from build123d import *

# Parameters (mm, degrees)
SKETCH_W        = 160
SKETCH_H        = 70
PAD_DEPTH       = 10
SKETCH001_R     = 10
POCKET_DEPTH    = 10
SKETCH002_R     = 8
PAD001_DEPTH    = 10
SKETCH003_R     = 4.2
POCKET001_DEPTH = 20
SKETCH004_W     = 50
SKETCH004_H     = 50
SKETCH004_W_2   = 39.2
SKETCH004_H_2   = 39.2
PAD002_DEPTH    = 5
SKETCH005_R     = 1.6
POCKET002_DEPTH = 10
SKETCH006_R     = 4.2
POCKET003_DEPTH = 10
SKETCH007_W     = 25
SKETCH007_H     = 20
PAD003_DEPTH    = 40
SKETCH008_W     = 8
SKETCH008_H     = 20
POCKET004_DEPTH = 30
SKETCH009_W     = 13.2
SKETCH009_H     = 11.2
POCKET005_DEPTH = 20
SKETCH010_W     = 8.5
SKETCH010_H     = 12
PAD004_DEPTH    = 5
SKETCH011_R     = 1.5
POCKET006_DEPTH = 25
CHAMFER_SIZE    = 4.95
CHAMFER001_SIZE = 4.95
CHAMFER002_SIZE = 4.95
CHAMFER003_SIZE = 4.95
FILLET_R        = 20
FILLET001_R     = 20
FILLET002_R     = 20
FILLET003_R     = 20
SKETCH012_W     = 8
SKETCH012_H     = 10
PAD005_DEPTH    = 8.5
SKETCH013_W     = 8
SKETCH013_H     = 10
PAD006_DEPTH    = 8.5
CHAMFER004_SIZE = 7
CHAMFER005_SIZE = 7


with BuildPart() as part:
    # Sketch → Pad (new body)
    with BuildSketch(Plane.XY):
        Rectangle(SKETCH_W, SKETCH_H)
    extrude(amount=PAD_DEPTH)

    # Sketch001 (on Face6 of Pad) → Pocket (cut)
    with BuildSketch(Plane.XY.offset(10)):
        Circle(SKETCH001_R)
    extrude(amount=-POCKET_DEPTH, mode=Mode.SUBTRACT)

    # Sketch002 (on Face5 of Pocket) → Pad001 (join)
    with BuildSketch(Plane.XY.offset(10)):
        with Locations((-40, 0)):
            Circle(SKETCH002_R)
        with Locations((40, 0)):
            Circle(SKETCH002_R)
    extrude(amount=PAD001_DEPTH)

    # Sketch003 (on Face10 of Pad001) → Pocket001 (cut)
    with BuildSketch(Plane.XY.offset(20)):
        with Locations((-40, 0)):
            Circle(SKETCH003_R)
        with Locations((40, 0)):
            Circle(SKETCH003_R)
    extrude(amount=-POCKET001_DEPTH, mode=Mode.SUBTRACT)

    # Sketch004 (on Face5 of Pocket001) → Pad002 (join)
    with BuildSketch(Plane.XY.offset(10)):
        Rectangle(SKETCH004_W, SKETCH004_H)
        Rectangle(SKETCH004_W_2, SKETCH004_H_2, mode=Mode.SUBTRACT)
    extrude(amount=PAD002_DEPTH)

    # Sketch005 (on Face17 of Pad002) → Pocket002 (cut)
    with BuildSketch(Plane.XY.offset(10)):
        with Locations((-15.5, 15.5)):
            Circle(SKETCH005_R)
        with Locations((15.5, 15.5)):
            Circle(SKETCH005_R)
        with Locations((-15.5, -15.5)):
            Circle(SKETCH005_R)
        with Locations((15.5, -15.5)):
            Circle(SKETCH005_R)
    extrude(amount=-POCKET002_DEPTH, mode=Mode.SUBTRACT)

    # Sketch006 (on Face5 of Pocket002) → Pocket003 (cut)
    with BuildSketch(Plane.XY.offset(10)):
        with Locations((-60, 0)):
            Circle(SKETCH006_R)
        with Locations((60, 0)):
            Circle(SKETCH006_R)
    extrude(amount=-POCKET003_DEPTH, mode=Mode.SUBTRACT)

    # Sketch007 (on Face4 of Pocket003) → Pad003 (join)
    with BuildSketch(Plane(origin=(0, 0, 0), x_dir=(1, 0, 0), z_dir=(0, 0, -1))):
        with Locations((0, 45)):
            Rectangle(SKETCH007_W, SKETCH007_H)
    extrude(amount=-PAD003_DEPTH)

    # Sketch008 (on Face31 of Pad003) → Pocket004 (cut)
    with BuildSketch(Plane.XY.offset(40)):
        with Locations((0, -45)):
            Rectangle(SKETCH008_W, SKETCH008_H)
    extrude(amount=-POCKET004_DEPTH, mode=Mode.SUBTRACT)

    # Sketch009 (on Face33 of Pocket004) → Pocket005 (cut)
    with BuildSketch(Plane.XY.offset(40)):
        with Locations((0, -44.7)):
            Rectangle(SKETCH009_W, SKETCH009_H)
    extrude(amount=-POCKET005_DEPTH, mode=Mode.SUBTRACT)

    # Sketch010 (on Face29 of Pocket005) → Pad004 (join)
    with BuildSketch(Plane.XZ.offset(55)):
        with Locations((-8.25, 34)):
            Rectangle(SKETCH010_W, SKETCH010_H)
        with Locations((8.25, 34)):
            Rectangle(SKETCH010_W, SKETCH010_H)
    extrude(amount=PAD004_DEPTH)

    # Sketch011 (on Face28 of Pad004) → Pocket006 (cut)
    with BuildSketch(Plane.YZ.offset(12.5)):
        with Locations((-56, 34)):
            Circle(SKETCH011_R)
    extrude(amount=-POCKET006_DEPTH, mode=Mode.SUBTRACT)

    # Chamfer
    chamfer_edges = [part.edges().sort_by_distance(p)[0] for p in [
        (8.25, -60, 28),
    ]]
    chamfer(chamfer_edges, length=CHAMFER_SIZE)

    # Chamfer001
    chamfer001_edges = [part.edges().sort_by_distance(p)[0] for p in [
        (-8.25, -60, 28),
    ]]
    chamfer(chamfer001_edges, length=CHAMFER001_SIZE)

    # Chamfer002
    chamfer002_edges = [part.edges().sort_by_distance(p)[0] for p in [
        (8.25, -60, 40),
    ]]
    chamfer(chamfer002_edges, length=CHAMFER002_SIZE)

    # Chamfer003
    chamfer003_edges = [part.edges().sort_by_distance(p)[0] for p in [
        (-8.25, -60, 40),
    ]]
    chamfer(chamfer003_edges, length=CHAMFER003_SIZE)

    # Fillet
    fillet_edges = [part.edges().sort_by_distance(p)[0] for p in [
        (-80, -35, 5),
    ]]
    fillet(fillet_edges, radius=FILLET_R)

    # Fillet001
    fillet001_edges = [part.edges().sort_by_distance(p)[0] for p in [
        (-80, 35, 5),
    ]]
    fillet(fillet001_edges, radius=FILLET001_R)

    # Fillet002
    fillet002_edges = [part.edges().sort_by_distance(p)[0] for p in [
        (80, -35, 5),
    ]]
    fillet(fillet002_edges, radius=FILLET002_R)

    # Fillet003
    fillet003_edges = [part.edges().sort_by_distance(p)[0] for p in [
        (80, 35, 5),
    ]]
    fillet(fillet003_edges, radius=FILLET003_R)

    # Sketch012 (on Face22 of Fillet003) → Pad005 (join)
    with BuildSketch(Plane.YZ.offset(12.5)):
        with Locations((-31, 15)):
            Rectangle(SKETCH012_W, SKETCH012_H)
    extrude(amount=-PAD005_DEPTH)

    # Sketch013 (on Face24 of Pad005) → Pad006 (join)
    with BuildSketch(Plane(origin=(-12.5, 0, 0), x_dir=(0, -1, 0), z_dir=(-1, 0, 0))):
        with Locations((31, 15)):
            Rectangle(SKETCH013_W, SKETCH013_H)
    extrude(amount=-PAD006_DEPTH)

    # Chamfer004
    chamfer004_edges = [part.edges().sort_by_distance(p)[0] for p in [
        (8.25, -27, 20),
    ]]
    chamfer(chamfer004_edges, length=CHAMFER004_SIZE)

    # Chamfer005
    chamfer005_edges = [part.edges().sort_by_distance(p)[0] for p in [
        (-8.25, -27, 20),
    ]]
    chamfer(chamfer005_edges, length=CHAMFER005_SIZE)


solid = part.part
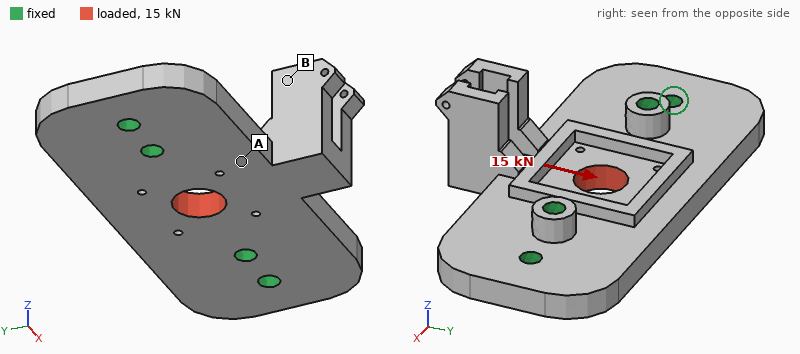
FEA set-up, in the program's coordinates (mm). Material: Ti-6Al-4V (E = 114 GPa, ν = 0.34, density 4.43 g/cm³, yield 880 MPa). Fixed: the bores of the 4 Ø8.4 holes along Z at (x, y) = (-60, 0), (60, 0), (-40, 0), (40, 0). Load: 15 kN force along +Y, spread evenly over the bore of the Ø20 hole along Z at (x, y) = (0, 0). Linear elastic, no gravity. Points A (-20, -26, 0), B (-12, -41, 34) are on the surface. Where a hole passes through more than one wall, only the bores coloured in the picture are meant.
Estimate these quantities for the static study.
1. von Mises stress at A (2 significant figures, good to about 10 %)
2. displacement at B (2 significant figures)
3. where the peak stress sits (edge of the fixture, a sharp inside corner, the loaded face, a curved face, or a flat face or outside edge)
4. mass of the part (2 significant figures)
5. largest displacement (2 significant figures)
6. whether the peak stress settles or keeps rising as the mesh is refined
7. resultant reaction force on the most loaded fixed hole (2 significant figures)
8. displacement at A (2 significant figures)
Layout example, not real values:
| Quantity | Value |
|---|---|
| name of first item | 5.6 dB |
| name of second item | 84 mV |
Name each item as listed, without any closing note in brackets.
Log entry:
| Quantity | Value |
|---|---|
| von Mises stress at A | 18 MPa |
| displacement at B | 10 µm |
| where the peak stress sits | edge of the fixture |
| mass of the part | 560 g |
| largest displacement | 15 µm |
| whether the peak stress settles or keeps rising as the mesh is refined | keeps rising |
| resultant reaction force on the most loaded fixed hole | 8.4 kN |
| displacement at A | 9.1 µm |
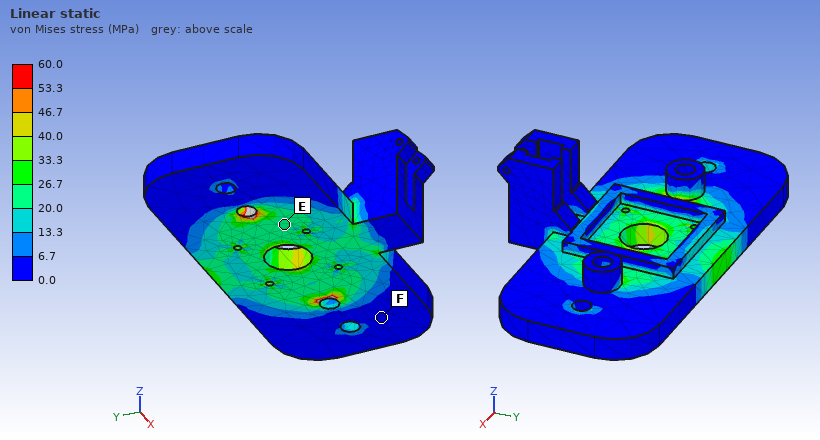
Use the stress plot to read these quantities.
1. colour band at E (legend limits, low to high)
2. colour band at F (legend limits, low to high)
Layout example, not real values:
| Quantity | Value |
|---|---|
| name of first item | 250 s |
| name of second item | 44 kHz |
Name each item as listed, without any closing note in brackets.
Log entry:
| Quantity | Value |
|---|---|
| colour band at E | 20.0 to 26.7 MPa |
| colour band at F | 0.0 to 6.7 MPa |
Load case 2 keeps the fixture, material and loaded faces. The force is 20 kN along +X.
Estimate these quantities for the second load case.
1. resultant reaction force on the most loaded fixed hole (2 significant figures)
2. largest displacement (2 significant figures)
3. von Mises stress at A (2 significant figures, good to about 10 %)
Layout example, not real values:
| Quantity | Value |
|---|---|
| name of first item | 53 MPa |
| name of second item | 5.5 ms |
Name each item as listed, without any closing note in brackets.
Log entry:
| Quantity | Value |
|---|---|
| resultant reaction force on the most loaded fixed hole | 7.7 kN |
| largest displacement | 9.7 µm |
| von Mises stress at A | 6.0 MPa |
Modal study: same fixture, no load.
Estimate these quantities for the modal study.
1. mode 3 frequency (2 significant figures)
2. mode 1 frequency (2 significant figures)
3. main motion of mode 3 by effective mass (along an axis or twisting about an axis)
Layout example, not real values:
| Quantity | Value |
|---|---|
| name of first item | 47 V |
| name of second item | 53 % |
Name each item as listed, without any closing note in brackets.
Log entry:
| Quantity | Value |
|---|---|
| mode 3 frequency | 5600 Hz |
| mode 1 frequency | 2200 Hz |
| main motion of mode 3 by effective mass | along Z |
